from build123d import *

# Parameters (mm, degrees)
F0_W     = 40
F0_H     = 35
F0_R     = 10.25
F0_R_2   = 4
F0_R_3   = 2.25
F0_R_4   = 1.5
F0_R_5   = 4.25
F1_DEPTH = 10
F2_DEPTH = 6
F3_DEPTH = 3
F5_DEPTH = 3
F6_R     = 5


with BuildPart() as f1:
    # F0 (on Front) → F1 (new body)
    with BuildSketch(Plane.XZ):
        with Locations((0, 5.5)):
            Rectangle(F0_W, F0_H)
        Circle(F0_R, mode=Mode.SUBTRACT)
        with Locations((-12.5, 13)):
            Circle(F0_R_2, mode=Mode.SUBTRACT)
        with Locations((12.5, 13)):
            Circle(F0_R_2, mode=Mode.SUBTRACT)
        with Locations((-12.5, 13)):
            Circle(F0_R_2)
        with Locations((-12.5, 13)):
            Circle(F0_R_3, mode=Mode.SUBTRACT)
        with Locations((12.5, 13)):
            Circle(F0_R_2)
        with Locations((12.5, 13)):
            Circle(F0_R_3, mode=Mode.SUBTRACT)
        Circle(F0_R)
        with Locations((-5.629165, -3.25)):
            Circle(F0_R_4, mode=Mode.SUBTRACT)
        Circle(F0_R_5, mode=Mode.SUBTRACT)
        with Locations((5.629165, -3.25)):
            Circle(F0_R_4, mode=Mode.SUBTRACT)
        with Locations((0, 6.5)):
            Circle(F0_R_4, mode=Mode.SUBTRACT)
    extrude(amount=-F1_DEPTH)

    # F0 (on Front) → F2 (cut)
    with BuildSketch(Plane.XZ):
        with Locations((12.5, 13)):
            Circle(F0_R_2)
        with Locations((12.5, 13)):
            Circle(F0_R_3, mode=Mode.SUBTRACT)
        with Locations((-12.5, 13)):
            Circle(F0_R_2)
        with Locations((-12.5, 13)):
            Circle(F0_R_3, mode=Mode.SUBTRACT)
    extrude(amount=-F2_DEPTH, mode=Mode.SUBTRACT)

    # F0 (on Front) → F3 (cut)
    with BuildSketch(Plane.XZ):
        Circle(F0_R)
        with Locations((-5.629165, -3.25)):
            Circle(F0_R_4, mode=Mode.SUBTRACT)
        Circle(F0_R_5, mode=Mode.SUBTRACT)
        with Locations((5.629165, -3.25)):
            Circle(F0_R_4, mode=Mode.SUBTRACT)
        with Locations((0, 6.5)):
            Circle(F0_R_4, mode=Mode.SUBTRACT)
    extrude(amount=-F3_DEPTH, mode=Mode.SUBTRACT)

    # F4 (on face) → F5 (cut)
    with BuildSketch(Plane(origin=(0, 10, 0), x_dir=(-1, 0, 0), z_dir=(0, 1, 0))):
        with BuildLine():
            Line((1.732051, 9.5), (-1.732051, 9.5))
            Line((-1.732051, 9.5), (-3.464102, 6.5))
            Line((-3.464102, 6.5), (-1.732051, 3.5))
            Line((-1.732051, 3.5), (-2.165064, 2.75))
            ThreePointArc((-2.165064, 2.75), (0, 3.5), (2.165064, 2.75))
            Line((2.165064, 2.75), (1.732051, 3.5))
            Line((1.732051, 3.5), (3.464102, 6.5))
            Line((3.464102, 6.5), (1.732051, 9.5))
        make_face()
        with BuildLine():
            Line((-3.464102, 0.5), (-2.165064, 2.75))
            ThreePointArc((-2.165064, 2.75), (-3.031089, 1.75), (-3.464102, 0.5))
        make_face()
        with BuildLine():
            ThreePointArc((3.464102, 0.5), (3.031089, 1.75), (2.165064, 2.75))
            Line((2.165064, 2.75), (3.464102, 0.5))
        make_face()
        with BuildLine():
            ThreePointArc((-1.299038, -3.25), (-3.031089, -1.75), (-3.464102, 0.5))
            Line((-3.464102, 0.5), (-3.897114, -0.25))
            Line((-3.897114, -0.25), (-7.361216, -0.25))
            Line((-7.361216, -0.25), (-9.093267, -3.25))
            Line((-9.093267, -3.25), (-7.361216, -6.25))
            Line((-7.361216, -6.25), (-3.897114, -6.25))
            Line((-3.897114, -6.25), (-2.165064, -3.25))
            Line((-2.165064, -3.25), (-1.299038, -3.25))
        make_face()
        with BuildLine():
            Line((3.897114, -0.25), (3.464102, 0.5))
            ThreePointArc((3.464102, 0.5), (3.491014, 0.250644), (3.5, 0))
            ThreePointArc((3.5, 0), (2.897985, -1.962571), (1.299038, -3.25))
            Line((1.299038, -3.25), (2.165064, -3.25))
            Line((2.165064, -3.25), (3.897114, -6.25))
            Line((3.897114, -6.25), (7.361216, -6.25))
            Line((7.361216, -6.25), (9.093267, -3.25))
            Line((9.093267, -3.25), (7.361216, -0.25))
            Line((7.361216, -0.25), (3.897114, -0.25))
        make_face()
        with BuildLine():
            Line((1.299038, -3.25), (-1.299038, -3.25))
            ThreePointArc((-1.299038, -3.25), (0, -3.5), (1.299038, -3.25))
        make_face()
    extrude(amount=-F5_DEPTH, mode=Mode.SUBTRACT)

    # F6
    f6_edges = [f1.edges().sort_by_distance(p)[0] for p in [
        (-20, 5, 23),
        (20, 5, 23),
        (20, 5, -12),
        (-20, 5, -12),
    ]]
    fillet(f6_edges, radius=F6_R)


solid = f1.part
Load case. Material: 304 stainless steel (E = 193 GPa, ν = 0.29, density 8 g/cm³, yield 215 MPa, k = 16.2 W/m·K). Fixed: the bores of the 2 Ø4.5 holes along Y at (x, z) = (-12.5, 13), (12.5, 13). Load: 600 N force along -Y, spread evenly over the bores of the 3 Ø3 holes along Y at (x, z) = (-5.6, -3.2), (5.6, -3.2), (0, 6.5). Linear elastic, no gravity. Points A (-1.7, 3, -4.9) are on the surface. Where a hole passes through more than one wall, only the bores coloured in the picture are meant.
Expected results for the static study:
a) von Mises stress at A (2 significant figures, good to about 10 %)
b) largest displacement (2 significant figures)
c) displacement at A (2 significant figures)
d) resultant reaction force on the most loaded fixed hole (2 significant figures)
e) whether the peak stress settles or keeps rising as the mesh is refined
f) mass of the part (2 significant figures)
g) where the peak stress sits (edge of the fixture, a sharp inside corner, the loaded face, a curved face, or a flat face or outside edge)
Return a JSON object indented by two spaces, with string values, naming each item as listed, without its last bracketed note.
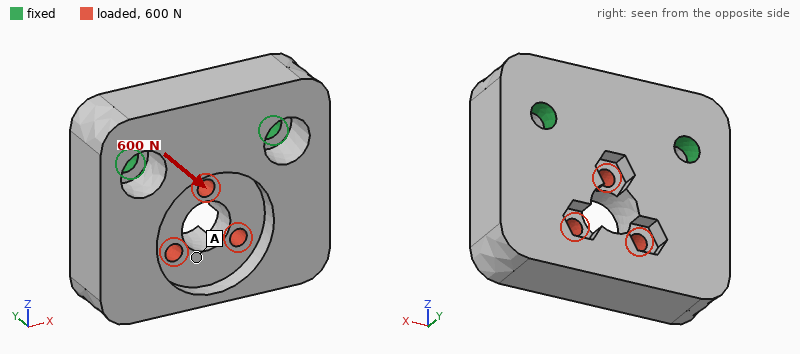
{
  "von Mises stress at A": "6.4 MPa",
  "largest displacement": "11 µm",
  "displacement at A": "8.1 µm",
  "resultant reaction force on the most loaded fixed hole": "330 N",
  "whether the peak stress settles or keeps rising as the mesh is refined": "keeps rising",
  "mass of the part": "91 g",
  "where the peak stress sits": "edge of the fixture"
}
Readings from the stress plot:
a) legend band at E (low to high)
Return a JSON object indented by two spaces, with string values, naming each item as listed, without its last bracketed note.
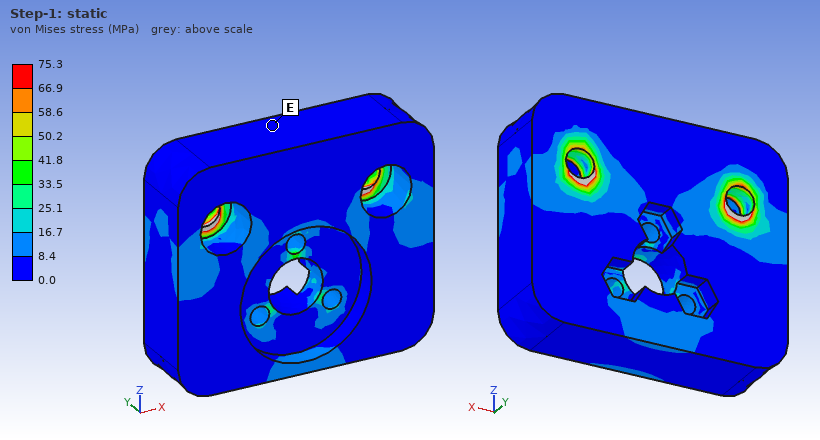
{
  "legend band at E": "0.0 to 8.4 MPa"
}
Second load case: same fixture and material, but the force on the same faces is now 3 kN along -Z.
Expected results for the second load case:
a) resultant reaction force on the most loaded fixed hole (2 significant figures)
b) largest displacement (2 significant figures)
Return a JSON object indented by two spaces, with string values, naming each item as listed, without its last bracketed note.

{
  "resultant reaction force on the most loaded fixed hole": "1.5 kN",
  "largest displacement": "12 µm"
}
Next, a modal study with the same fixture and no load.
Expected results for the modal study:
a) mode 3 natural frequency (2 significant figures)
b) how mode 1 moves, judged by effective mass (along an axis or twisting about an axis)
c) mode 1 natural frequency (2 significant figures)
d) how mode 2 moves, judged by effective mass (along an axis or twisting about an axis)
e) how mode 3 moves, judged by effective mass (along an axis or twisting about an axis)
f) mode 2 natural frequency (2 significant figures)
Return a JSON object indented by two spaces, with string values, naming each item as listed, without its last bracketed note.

{
  "mode 3 natural frequency": "16 kHz",
  "how mode 1 moves, judged by effective mass": "along Y",
  "mode 1 natural frequency": "5800 Hz",
  "how mode 2 moves, judged by effective mass": "twisting about Z",
  "how mode 3 moves, judged by effective mass": "along X",
  "mode 2 natural frequency": "12 kHz"
}
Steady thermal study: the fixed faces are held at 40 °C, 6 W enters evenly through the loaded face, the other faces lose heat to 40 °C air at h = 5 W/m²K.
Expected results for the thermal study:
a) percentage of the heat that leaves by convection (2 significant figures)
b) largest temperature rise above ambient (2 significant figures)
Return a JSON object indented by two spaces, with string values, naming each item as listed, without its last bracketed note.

{
  "percentage of the heat that leaves by convection": "5.2 %",
  "largest temperature rise above ambient": "33 K"
}
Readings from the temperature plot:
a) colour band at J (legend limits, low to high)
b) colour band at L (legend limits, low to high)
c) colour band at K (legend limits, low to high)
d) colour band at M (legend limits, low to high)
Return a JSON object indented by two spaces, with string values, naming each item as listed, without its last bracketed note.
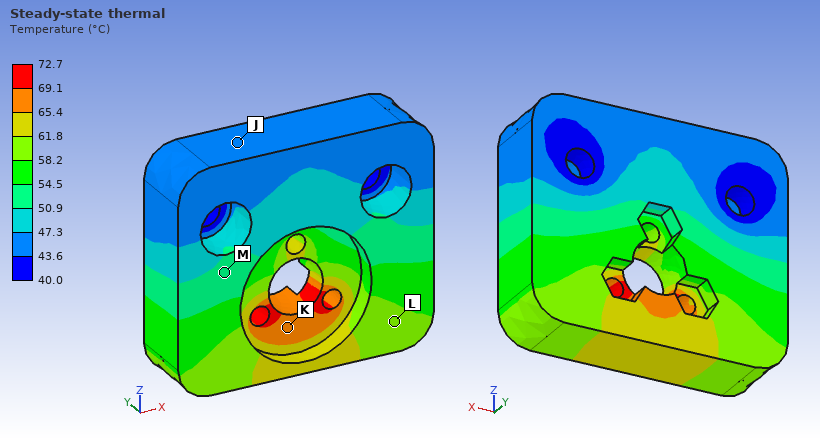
{
  "colour band at J": "43.6 to 47.3 °C",
  "colour band at L": "58.2 to 61.8 °C",
  "colour band at K": "65.4 to 69.1 °C",
  "colour band at M": "50.9 to 54.5 °C"
}
